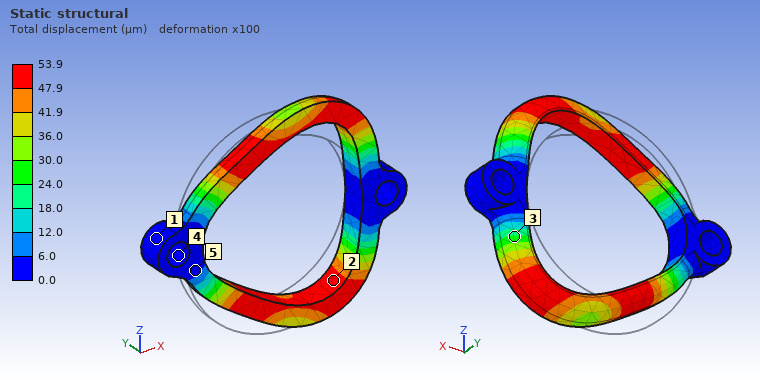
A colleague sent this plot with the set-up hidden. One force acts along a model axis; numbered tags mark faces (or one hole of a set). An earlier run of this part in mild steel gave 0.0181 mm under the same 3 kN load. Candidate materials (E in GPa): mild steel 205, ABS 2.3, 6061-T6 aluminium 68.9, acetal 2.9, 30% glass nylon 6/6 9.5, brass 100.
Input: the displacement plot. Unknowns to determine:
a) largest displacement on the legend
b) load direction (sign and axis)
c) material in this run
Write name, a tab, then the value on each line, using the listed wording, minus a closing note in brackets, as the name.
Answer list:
largest displacement on the legend	53.9 µm
load direction	+X
material in this run	6061-T6 aluminium
